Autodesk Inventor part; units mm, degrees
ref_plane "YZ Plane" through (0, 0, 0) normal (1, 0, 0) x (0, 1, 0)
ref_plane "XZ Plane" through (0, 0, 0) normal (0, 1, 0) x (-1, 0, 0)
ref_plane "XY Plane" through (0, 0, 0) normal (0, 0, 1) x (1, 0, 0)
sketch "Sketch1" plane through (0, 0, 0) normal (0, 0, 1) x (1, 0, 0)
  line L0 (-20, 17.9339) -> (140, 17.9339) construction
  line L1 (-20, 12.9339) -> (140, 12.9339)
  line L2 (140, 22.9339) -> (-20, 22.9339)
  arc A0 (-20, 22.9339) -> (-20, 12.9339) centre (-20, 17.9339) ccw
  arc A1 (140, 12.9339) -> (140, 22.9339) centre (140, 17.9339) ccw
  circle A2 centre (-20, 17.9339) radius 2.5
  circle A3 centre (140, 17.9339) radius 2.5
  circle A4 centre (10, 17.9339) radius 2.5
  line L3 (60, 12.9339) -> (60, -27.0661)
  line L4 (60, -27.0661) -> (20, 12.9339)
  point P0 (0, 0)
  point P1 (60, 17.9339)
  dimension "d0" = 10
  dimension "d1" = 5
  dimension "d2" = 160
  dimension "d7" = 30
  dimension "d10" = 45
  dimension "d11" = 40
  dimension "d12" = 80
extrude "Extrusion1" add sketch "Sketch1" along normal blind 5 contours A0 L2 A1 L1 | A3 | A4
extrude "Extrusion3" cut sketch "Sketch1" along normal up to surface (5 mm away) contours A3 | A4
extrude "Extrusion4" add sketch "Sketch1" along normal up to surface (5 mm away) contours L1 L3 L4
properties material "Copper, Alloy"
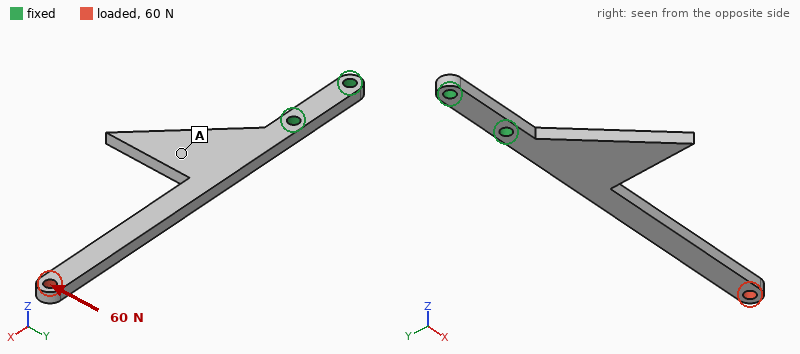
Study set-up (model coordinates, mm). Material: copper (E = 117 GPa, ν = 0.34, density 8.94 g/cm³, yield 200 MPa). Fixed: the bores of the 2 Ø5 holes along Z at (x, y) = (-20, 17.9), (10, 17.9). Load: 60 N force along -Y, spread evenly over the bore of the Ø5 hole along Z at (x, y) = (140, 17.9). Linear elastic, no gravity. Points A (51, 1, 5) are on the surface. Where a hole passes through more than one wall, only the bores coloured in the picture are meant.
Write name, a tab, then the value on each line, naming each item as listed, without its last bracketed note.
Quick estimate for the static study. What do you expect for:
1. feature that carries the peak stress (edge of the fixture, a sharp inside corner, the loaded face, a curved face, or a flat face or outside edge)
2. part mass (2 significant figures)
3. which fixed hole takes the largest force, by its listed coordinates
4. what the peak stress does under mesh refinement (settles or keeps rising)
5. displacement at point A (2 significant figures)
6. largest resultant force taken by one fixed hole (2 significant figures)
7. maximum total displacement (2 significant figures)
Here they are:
feature that carries the peak stress	edge of the fixture
part mass	110 g
which fixed hole takes the largest force, by its listed coordinates	(10, 17.9)
what the peak stress does under mesh refinement	keeps rising
displacement at point A	0.098 mm
largest resultant force taken by one fixed hole	100 N
maximum total displacement	0.62 mm
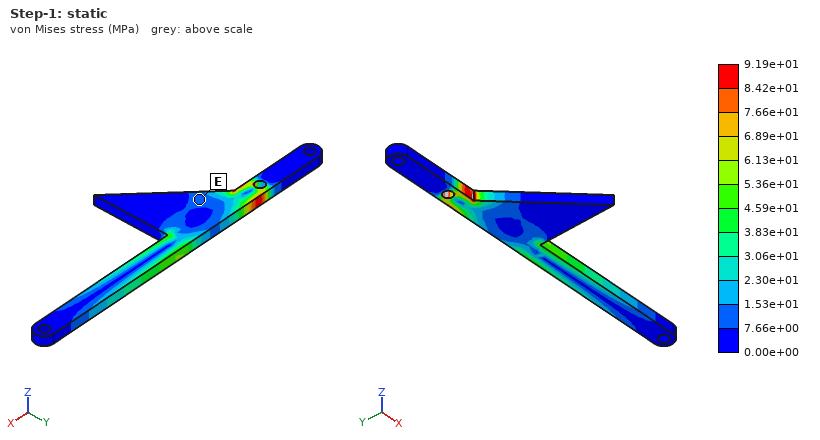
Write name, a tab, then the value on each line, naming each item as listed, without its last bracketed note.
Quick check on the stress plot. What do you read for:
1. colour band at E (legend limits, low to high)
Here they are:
colour band at E	7.66e+00 to 1.53e+01 MPa
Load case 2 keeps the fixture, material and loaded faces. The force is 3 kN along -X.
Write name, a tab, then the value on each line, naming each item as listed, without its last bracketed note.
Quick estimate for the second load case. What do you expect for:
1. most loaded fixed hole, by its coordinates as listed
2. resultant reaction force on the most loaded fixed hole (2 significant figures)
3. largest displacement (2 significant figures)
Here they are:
most loaded fixed hole, by its coordinates as listed	(10, 17.9)
resultant reaction force on the most loaded fixed hole	3.0 kN
largest displacement	0.15 mm
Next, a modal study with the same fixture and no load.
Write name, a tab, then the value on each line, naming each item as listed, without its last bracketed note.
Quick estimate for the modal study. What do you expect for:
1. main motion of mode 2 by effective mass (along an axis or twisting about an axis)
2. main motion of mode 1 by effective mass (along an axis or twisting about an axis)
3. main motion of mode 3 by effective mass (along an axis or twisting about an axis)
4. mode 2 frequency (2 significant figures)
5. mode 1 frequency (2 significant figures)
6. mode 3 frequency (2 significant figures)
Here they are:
main motion of mode 2 by effective mass	along Y
main motion of mode 1 by effective mass	along Z
main motion of mode 3 by effective mass	along Z
mode 2 frequency	400 Hz
mode 1 frequency	190 Hz
mode 3 frequency	750 Hz
